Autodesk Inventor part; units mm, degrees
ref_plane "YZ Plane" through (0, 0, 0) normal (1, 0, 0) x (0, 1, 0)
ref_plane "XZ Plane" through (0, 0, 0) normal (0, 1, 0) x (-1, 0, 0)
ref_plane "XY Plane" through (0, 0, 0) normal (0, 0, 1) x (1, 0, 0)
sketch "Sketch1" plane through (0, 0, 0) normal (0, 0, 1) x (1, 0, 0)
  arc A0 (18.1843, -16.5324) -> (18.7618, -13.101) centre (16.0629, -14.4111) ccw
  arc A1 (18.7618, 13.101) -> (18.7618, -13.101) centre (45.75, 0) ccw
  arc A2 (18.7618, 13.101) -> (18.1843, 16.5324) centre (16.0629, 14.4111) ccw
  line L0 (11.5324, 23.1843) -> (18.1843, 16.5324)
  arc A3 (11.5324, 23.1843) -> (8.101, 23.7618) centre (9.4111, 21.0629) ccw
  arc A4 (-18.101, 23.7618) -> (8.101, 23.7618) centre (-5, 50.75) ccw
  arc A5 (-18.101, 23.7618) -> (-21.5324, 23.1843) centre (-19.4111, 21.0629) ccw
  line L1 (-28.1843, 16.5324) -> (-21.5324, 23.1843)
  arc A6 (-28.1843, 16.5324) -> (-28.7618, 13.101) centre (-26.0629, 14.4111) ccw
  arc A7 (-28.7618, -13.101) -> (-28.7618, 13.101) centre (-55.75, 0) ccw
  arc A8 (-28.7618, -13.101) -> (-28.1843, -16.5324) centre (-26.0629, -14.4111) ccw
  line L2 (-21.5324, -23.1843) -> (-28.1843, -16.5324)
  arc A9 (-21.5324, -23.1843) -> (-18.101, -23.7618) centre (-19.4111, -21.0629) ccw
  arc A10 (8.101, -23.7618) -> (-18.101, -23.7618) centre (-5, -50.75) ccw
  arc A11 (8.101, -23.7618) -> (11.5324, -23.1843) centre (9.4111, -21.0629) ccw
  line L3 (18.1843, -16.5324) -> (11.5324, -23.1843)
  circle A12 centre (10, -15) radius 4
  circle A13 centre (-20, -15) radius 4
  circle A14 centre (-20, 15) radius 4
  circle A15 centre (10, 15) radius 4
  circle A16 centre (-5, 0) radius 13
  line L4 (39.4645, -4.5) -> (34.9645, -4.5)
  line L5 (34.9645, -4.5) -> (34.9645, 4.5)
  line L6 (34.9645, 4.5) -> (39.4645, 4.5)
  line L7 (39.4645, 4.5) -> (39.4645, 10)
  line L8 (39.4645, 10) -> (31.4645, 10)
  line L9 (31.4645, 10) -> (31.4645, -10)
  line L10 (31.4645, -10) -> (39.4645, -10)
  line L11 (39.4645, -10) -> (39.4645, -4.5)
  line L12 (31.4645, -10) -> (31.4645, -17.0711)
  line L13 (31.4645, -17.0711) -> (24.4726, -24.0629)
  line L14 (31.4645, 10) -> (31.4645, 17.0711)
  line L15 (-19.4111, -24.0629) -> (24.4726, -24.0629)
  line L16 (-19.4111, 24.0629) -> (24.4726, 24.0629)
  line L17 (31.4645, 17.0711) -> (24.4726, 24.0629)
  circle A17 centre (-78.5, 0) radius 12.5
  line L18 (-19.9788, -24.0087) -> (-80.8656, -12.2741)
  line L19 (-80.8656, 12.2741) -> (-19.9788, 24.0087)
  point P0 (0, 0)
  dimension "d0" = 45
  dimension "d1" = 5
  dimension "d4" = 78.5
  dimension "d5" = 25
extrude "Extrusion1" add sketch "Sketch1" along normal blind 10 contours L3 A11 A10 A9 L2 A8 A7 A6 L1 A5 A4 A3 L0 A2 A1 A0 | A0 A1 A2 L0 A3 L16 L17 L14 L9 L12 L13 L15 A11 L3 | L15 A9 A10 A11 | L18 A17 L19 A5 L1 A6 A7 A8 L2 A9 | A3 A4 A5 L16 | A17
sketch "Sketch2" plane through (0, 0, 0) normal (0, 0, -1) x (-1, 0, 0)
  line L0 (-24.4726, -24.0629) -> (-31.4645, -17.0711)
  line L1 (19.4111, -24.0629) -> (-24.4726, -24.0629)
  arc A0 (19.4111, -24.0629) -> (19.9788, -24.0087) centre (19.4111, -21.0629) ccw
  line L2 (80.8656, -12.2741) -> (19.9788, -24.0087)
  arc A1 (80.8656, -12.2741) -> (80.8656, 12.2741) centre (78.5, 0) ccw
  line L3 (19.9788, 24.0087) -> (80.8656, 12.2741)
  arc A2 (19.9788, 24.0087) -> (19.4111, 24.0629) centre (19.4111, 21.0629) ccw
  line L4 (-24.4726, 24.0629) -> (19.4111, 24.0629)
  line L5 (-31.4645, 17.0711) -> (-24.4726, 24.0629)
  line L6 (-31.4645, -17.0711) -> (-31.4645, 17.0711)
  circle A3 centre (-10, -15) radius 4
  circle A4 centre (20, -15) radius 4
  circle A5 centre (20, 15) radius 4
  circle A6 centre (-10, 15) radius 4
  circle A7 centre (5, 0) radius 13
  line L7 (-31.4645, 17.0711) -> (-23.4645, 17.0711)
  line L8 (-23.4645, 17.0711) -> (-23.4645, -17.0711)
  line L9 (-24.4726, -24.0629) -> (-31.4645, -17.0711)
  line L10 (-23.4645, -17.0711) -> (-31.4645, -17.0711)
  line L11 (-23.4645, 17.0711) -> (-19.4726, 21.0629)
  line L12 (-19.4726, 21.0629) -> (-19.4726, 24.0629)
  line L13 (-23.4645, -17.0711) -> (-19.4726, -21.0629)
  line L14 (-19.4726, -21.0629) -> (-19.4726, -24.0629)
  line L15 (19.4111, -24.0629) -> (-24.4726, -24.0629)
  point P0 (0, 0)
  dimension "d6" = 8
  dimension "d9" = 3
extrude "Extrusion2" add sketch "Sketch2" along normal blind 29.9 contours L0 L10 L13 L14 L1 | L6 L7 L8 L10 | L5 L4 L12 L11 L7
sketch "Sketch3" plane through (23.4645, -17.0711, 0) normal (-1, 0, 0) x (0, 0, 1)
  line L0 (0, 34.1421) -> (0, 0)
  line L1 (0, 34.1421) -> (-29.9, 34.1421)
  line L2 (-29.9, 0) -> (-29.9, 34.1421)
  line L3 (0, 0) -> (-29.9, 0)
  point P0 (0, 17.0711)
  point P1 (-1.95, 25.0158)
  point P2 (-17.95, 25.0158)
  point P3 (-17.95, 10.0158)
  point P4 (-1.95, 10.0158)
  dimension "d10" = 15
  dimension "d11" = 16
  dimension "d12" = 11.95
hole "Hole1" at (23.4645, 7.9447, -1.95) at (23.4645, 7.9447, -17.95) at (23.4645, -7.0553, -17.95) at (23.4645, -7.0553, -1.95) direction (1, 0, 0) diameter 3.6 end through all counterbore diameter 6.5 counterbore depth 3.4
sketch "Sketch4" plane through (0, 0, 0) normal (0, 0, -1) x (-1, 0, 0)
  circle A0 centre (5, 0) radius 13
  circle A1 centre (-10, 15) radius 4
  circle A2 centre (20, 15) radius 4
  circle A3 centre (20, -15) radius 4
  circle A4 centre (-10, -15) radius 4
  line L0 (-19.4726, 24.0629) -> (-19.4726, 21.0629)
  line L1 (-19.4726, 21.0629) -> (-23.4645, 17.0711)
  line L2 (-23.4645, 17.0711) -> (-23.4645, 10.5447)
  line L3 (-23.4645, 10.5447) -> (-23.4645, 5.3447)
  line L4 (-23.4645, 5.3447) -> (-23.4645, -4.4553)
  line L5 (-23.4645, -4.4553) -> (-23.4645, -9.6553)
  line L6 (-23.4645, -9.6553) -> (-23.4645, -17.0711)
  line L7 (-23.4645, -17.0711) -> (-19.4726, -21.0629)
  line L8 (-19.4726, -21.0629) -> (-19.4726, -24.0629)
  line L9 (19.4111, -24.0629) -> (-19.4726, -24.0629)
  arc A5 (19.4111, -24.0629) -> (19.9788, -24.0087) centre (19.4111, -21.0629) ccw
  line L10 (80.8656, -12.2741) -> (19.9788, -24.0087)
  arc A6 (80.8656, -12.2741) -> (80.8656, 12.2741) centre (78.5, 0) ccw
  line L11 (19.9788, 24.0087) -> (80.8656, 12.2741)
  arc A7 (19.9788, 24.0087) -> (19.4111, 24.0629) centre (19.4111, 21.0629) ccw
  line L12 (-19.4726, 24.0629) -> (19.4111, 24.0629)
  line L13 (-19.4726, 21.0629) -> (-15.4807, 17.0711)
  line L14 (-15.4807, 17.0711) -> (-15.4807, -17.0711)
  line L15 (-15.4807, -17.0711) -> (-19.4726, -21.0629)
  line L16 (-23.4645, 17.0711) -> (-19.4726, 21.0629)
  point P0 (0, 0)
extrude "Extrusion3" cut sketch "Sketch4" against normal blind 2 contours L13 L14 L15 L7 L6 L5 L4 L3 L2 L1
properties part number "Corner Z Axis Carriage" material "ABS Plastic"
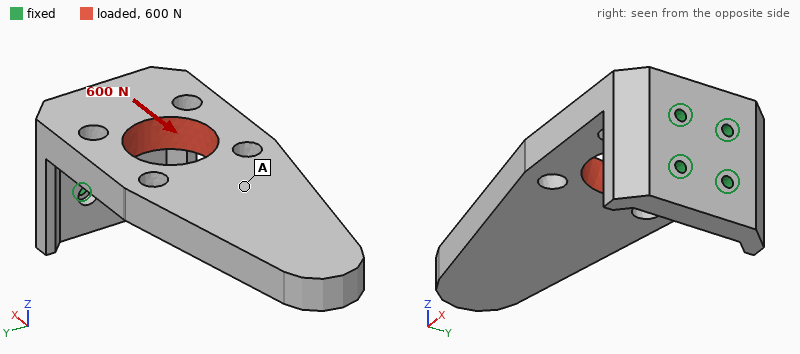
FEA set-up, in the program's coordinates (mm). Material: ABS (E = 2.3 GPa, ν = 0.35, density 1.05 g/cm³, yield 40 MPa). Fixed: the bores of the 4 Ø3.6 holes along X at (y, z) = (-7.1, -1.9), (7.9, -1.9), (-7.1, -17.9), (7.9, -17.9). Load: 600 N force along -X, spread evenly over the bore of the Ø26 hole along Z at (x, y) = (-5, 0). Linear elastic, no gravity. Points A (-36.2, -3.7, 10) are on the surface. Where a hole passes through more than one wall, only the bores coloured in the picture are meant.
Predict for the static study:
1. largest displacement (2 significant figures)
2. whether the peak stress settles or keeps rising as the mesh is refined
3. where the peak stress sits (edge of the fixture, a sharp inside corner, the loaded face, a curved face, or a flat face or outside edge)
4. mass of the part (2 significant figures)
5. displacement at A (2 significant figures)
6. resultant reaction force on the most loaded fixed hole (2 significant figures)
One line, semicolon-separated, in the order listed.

0.82 mm; keeps rising; edge of the fixture; 53 g; 0.46 mm; 390 N
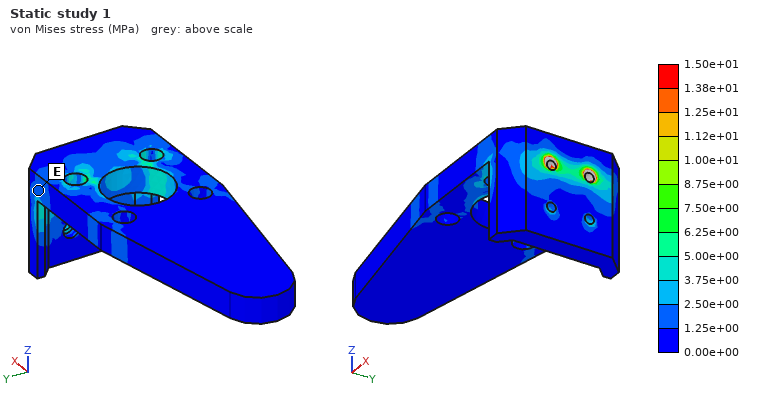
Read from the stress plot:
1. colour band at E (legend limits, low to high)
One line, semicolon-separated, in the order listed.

1.25e+00 to 2.50e+00 MPa
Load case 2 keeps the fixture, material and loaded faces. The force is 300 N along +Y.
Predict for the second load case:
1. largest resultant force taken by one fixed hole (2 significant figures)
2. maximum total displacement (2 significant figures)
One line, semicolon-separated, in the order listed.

510 N; 1.2 mm
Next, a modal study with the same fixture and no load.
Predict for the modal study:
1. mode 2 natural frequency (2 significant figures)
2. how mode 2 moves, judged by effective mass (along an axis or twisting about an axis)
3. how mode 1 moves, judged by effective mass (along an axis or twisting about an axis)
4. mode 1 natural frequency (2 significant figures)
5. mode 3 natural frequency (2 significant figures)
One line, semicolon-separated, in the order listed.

360 Hz; along Y; along Z; 140 Hz; 910 Hz
